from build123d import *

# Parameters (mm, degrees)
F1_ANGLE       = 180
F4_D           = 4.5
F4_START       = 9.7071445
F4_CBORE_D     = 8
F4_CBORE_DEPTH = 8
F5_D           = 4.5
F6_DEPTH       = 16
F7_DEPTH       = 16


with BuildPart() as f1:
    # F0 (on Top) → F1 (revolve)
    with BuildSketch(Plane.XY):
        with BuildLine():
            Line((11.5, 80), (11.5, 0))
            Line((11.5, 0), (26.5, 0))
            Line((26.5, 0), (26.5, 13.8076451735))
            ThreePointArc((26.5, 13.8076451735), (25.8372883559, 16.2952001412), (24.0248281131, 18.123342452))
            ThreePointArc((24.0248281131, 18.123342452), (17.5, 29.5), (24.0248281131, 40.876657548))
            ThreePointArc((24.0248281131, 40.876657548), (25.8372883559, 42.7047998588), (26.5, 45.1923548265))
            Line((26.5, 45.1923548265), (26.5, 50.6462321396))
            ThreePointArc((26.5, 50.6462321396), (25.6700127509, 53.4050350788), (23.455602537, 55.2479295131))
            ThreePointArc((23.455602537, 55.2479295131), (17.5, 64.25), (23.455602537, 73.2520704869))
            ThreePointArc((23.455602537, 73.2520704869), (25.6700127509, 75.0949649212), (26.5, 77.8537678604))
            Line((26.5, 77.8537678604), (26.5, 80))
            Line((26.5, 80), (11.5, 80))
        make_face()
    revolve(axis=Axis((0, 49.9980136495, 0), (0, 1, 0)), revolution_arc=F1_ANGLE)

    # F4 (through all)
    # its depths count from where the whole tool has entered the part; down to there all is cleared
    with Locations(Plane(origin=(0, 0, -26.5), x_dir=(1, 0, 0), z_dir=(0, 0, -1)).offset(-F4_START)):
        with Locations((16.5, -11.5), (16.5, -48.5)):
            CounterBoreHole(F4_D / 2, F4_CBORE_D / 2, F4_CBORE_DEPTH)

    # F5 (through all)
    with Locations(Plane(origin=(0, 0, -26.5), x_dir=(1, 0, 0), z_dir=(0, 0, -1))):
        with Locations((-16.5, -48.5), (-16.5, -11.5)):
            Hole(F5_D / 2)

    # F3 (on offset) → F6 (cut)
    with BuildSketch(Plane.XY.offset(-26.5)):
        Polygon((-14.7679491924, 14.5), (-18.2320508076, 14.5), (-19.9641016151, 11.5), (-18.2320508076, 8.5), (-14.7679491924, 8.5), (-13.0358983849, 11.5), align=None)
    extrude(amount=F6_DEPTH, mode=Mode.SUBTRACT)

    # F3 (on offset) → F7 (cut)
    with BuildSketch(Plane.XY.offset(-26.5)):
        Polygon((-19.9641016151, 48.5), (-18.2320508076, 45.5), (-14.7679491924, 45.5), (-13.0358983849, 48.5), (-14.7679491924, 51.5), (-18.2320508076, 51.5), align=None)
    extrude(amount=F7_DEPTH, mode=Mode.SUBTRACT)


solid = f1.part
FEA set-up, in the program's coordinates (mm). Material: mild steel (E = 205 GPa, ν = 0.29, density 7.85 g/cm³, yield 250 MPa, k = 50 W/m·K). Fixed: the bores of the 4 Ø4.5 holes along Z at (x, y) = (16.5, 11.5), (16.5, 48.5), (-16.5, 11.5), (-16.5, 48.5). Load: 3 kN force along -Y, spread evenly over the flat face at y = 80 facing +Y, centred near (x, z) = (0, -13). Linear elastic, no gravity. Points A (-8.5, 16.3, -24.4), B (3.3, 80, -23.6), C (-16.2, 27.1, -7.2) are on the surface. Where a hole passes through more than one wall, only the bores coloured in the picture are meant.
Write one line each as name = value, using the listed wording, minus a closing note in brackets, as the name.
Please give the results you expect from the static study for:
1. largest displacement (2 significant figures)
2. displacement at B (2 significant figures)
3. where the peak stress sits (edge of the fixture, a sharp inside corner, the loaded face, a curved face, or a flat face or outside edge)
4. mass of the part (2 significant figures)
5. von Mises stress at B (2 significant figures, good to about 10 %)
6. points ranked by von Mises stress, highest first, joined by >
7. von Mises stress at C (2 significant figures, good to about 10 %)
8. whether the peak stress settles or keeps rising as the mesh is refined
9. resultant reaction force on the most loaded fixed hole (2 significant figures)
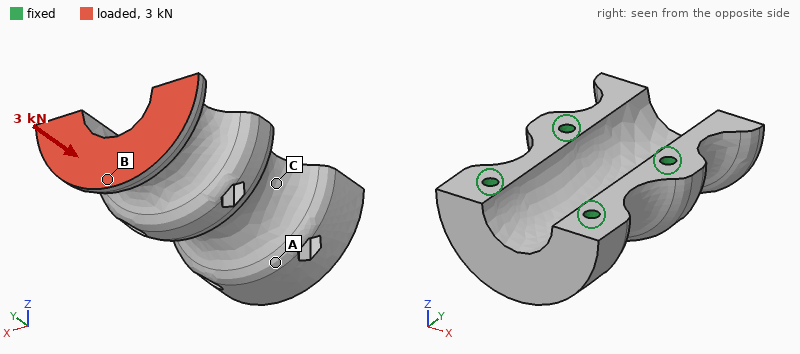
largest displacement = 8.1 µm
displacement at B = 7.4 µm
where the peak stress sits = edge of the fixture
mass of the part = 370 g
von Mises stress at B = 8.8 MPa
points ranked by von Mises stress, highest first, joined by > = B > C > A
von Mises stress at C = 5.2 MPa
whether the peak stress settles or keeps rising as the mesh is refined = keeps rising
resultant reaction force on the most loaded fixed hole = 1.1 kN
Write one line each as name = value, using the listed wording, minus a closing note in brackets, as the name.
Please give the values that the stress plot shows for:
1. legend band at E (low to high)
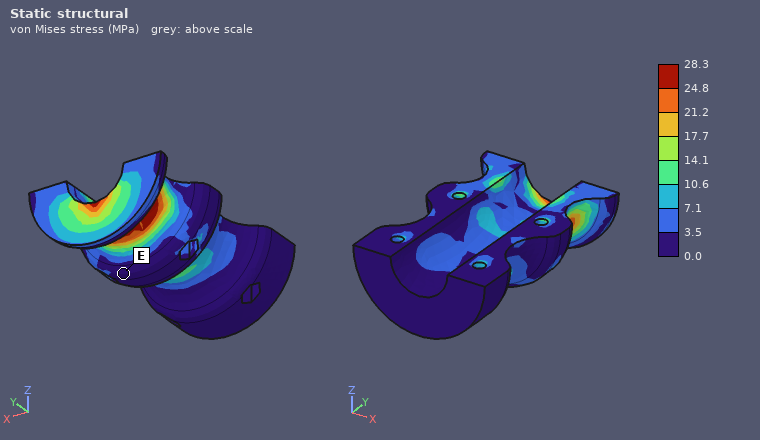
legend band at E = 0.0 to 3.5 MPa
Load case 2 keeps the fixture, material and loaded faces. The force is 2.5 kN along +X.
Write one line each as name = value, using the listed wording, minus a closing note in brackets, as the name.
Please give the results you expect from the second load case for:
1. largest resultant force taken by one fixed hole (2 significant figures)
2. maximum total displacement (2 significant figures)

largest resultant force taken by one fixed hole = 2.6 kN
maximum total displacement = 19 µm
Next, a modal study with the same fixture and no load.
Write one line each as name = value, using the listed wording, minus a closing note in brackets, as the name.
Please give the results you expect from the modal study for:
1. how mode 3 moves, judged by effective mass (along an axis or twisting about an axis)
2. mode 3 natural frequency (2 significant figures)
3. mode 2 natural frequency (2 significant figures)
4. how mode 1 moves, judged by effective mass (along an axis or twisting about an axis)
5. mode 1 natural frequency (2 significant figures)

how mode 3 moves, judged by effective mass = along X
mode 3 natural frequency = 13 kHz
mode 2 natural frequency = 8000 Hz
how mode 1 moves, judged by effective mass = along Z
mode 1 natural frequency = 7200 Hz
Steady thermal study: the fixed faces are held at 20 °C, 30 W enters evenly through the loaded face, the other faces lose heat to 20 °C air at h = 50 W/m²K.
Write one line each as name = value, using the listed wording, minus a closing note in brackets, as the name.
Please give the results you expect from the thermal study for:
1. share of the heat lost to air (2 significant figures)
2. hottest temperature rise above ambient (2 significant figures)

share of the heat lost to air = 21 %
hottest temperature rise above ambient = 46 K
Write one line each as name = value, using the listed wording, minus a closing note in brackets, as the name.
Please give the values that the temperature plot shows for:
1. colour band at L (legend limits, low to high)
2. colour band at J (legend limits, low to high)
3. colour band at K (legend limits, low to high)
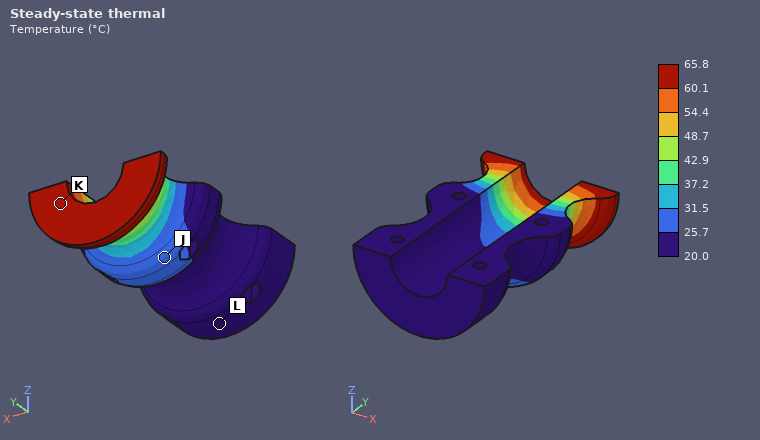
colour band at L = 20.0 to 25.7 °C
colour band at J = 25.7 to 31.5 °C
colour band at K = 60.1 to 65.8 °C
